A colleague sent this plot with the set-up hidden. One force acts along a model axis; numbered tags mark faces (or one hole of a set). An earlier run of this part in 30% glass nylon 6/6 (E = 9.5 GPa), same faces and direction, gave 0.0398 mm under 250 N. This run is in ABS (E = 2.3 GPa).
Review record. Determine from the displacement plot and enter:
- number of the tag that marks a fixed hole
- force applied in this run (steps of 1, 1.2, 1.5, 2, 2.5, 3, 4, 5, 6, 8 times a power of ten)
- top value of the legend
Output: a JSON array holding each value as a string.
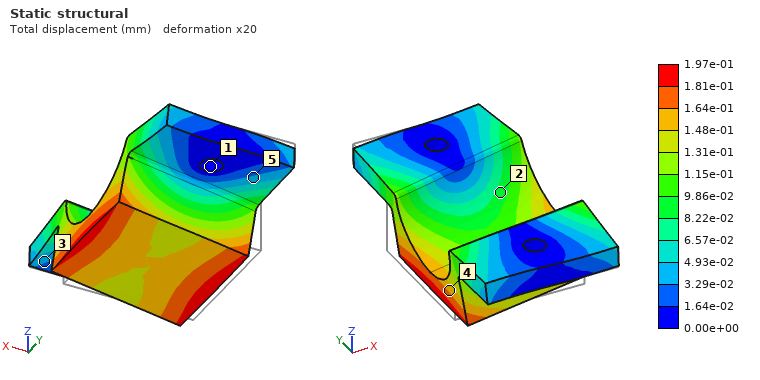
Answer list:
["1", "300 N", "1.97e-01 mm"]
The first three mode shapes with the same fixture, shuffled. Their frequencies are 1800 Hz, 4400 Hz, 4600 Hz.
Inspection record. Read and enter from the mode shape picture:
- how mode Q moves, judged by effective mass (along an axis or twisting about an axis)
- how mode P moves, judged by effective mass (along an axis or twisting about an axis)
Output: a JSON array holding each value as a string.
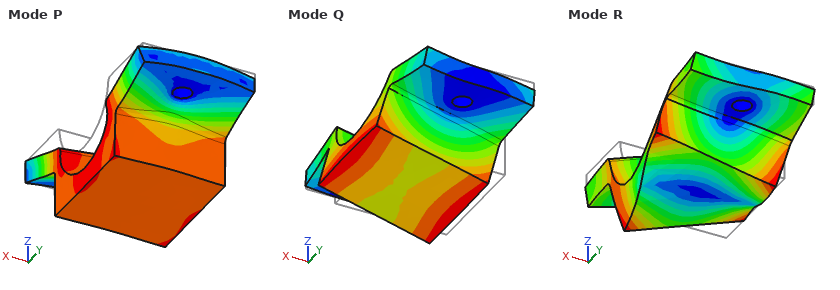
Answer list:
["along X", "along Z"]
